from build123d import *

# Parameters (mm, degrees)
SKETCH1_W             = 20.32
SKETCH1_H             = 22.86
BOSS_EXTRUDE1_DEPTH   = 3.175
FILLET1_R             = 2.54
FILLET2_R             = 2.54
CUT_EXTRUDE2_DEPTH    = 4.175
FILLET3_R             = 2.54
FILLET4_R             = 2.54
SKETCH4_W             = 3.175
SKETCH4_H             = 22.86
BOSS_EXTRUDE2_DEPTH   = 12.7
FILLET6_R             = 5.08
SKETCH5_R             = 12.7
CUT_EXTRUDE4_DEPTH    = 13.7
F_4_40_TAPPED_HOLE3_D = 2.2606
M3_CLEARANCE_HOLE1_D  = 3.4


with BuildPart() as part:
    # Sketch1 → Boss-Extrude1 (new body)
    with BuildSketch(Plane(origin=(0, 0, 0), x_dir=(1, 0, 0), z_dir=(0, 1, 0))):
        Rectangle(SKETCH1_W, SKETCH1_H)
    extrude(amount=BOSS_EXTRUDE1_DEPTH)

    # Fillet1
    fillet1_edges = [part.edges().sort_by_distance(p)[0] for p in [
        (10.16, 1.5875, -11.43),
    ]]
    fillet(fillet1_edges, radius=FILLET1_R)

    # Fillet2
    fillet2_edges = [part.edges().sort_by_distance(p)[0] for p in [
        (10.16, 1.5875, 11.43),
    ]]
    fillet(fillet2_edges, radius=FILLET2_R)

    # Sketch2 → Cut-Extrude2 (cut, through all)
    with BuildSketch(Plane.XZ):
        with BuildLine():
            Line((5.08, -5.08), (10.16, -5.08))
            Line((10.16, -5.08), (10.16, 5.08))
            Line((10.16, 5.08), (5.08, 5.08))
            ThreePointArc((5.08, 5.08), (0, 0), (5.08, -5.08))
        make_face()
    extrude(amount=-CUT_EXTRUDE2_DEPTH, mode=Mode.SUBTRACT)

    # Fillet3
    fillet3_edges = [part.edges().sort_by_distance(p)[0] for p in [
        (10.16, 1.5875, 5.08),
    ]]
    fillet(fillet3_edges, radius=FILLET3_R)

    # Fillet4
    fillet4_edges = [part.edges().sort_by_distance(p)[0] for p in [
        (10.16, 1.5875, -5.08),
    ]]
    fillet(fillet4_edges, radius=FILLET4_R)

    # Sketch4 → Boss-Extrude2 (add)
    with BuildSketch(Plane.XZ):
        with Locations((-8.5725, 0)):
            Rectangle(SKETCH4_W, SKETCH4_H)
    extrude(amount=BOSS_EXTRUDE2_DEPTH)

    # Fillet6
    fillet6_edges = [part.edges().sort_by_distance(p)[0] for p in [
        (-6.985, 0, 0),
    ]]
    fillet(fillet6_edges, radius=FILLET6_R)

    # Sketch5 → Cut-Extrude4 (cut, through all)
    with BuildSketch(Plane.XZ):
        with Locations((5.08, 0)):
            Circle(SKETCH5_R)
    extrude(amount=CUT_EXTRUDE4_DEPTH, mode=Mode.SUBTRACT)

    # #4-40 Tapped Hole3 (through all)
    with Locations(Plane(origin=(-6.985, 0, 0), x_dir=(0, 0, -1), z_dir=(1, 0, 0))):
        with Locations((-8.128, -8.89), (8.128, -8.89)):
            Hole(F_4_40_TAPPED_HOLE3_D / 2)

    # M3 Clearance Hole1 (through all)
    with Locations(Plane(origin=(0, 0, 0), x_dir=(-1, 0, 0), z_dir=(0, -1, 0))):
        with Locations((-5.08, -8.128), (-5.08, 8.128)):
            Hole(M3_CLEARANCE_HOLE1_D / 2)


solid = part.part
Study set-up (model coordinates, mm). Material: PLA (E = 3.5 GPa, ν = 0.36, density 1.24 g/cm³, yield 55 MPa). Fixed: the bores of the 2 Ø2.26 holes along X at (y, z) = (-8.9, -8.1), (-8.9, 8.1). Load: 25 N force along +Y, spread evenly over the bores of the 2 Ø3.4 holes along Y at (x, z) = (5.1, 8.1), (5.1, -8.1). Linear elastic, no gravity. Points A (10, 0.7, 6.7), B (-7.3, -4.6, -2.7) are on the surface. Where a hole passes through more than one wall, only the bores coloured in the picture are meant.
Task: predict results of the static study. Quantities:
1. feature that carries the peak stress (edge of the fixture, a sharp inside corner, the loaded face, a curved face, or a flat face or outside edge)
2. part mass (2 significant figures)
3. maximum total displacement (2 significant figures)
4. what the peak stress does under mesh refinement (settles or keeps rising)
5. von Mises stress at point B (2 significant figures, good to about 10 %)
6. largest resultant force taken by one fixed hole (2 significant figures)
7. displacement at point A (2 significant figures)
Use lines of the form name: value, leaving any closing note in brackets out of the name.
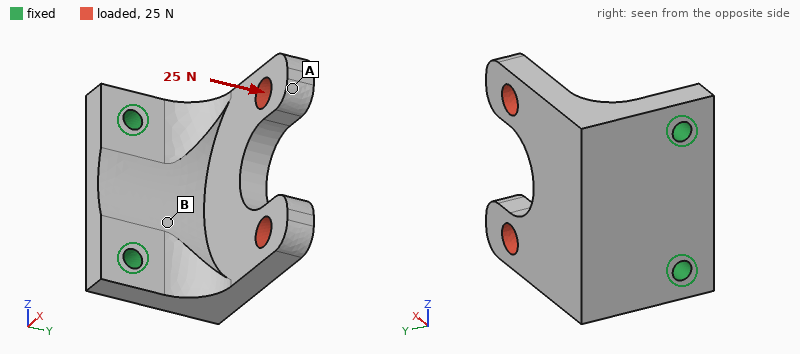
feature that carries the peak stress: edge of the fixture
part mass: 2.5 g
maximum total displacement: 0.41 mm
what the peak stress does under mesh refinement: keeps rising
von Mises stress at point B: 5.9 MPa
largest resultant force taken by one fixed hole: 13 N
displacement at point A: 0.39 mm
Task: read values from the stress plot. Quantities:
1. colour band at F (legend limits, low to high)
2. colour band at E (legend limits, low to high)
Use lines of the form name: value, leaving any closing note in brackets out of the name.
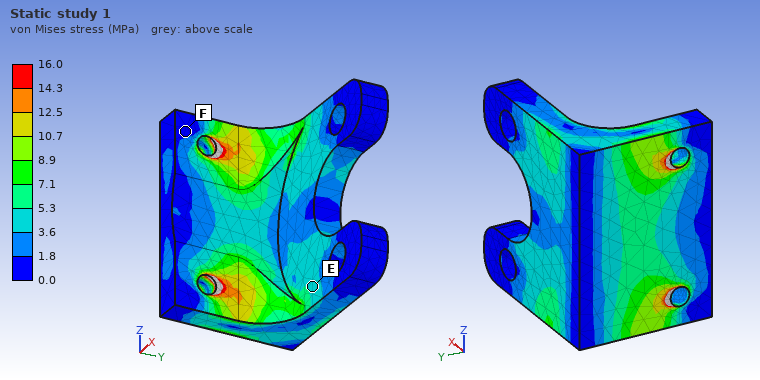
colour band at F: 0.0 to 1.8 MPa
colour band at E: 3.6 to 5.3 MPa
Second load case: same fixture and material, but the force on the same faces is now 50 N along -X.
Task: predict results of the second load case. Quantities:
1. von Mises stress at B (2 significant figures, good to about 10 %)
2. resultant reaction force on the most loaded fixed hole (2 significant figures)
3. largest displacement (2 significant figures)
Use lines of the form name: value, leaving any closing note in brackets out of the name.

von Mises stress at B: 5.2 MPa
resultant reaction force on the most loaded fixed hole: 25 N
largest displacement: 0.30 mm
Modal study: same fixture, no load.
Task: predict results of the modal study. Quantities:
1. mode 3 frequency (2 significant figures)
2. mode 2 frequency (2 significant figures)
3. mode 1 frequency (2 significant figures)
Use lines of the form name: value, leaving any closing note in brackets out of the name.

mode 3 frequency: 4500 Hz
mode 2 frequency: 3000 Hz
mode 1 frequency: 1800 Hz
